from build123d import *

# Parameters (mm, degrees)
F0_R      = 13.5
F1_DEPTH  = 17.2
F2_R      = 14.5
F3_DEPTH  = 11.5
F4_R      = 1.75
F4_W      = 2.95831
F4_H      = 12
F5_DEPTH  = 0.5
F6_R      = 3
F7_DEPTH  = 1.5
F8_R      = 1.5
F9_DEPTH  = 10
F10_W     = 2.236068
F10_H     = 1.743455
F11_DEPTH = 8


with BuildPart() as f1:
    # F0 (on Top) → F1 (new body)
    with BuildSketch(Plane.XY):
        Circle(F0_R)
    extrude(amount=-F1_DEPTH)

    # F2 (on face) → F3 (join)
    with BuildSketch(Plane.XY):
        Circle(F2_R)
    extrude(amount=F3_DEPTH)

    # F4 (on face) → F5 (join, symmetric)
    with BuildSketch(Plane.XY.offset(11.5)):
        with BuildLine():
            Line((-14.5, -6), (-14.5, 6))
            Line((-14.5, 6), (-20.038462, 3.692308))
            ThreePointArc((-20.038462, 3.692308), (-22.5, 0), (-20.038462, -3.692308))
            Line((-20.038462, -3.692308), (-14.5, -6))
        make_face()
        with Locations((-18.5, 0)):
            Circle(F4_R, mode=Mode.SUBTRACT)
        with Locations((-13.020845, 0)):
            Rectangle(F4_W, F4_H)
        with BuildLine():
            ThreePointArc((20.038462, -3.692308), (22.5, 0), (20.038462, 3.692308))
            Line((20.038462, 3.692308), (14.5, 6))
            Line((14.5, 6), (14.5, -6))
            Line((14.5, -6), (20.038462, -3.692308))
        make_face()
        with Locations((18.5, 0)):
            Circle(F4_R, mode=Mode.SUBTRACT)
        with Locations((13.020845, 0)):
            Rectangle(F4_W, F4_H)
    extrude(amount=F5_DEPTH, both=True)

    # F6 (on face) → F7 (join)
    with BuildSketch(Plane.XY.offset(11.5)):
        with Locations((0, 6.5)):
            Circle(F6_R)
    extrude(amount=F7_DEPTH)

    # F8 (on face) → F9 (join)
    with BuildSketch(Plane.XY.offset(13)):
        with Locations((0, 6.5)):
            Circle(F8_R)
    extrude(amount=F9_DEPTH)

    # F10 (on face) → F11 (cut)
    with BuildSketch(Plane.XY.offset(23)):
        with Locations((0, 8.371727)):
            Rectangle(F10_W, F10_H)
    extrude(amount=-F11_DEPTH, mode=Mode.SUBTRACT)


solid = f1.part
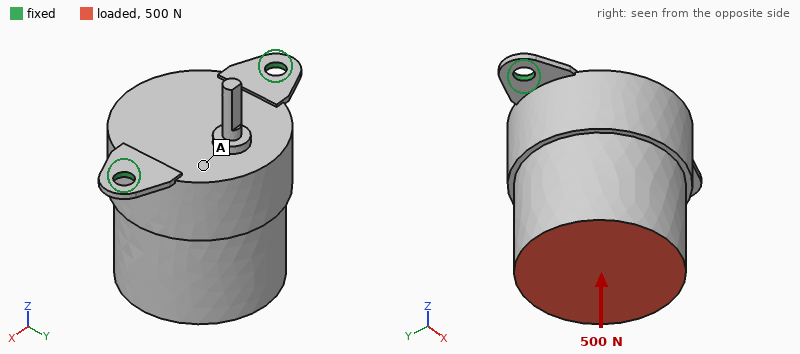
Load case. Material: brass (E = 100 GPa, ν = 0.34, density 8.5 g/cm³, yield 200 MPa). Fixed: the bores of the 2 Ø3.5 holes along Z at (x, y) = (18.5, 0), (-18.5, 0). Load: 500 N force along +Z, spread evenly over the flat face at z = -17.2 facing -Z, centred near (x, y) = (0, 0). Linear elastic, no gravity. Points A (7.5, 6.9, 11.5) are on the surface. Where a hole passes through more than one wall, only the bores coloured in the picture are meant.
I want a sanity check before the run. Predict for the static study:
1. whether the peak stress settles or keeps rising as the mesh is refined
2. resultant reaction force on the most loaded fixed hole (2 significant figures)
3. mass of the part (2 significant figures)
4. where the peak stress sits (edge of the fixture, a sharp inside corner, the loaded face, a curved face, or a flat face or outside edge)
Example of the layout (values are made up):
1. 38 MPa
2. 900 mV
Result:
1. keeps rising
2. 290 N
3. 150 g
4. edge of the fixture
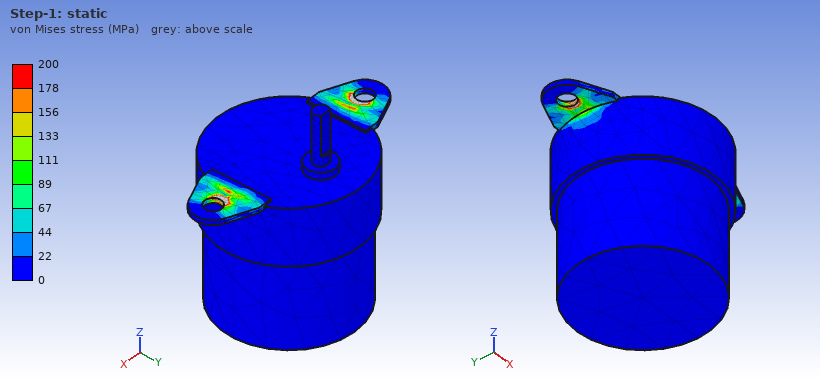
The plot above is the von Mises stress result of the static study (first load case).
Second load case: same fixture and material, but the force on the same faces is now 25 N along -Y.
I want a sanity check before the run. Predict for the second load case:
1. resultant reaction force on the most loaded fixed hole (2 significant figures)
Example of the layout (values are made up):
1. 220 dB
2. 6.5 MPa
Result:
1. 13 N
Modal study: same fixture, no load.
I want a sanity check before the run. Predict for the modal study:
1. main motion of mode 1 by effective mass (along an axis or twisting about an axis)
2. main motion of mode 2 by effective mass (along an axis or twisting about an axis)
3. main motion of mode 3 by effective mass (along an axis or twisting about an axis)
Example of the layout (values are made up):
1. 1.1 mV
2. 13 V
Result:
1. along Y
2. along X
3. along Z
